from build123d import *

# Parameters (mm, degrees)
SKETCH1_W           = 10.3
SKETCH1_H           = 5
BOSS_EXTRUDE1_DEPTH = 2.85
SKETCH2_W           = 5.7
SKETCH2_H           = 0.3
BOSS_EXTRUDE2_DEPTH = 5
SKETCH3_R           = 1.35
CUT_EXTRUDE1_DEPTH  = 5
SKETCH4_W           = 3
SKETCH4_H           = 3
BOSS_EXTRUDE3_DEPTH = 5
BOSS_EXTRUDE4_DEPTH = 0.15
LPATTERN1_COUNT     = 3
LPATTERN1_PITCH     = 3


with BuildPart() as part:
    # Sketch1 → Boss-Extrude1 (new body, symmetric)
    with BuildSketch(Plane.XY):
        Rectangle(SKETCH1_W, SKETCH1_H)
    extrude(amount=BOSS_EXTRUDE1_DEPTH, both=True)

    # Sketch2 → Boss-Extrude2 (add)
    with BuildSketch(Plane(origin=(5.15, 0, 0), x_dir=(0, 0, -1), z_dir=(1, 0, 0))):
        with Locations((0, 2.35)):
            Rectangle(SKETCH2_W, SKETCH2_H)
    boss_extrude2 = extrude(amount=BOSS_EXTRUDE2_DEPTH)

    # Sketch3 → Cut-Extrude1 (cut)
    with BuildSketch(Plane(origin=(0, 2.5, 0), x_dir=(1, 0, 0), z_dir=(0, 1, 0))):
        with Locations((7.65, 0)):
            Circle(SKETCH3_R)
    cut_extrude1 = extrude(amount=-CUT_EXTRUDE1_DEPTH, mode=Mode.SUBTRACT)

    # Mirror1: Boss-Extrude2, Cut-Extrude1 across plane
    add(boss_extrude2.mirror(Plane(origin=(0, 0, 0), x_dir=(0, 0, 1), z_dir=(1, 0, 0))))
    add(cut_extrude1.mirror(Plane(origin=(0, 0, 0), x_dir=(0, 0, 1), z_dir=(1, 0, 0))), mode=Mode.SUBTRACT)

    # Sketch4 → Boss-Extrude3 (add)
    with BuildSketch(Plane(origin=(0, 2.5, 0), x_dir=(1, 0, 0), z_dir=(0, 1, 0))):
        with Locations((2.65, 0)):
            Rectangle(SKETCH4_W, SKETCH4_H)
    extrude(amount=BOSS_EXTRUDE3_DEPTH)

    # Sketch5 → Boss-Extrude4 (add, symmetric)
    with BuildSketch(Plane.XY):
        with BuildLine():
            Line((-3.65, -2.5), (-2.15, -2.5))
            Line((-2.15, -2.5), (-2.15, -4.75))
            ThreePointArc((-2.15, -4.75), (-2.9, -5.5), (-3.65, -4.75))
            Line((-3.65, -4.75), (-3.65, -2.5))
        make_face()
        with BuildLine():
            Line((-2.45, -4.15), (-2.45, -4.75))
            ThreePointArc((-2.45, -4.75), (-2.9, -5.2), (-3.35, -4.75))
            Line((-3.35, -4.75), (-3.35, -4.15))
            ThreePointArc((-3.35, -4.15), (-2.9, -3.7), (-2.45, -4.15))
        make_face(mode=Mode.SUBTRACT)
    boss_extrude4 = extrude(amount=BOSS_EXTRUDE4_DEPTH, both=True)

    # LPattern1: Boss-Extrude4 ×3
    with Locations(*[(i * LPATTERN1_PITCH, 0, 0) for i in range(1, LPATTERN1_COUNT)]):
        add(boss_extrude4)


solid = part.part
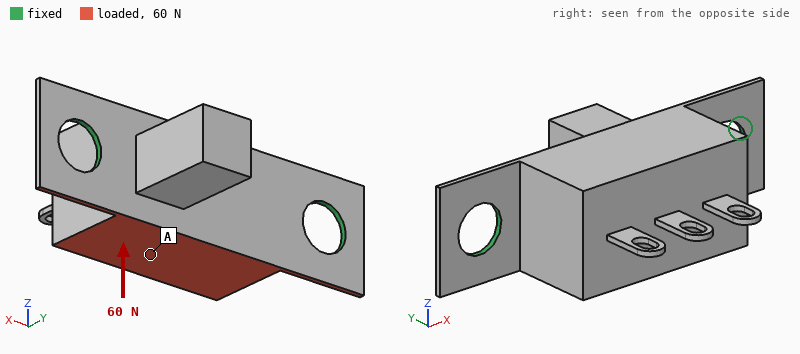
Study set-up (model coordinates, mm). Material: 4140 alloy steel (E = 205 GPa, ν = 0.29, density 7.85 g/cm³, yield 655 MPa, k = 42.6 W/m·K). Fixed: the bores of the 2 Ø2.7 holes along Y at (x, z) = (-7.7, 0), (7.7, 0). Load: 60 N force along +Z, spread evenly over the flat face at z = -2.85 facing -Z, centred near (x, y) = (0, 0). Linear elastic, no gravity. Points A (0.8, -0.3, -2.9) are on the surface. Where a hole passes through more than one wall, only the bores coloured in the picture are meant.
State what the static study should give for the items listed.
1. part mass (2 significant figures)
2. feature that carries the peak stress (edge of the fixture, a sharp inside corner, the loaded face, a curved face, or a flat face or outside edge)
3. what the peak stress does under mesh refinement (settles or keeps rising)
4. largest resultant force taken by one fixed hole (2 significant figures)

2.8 g
edge of the fixture
keeps rising
31 N
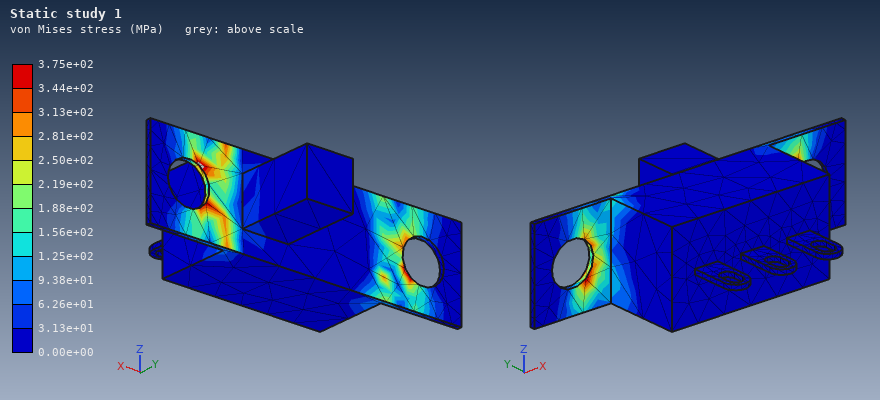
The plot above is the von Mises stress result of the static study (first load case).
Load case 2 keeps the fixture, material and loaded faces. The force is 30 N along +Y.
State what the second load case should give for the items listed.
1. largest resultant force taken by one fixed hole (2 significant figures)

18 N
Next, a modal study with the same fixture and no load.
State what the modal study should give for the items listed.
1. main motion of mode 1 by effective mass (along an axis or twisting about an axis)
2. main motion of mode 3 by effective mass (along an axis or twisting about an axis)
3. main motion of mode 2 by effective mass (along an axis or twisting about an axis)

along Z
along X
along Y
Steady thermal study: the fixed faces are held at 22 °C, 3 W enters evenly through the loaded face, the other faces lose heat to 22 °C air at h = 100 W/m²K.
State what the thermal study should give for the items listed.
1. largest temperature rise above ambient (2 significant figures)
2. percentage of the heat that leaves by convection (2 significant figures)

33 K
32 %
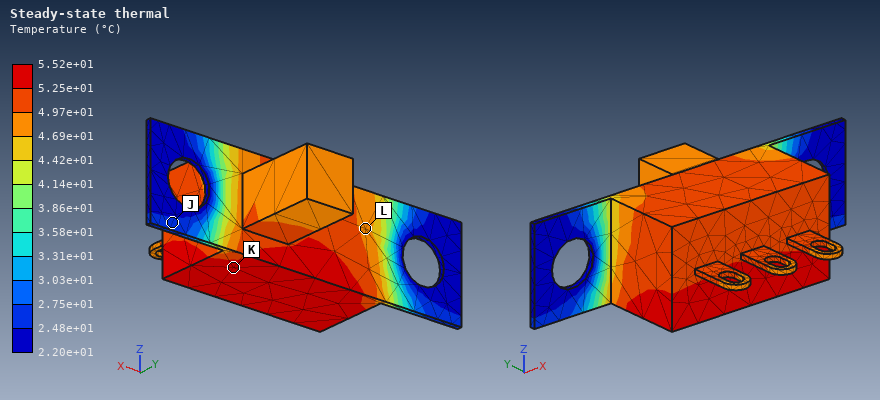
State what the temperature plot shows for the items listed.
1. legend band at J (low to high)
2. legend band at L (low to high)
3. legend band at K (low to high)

2.48e+01 to 2.75e+01 °C
4.69e+01 to 4.97e+01 °C
5.25e+01 to 5.52e+01 °C
